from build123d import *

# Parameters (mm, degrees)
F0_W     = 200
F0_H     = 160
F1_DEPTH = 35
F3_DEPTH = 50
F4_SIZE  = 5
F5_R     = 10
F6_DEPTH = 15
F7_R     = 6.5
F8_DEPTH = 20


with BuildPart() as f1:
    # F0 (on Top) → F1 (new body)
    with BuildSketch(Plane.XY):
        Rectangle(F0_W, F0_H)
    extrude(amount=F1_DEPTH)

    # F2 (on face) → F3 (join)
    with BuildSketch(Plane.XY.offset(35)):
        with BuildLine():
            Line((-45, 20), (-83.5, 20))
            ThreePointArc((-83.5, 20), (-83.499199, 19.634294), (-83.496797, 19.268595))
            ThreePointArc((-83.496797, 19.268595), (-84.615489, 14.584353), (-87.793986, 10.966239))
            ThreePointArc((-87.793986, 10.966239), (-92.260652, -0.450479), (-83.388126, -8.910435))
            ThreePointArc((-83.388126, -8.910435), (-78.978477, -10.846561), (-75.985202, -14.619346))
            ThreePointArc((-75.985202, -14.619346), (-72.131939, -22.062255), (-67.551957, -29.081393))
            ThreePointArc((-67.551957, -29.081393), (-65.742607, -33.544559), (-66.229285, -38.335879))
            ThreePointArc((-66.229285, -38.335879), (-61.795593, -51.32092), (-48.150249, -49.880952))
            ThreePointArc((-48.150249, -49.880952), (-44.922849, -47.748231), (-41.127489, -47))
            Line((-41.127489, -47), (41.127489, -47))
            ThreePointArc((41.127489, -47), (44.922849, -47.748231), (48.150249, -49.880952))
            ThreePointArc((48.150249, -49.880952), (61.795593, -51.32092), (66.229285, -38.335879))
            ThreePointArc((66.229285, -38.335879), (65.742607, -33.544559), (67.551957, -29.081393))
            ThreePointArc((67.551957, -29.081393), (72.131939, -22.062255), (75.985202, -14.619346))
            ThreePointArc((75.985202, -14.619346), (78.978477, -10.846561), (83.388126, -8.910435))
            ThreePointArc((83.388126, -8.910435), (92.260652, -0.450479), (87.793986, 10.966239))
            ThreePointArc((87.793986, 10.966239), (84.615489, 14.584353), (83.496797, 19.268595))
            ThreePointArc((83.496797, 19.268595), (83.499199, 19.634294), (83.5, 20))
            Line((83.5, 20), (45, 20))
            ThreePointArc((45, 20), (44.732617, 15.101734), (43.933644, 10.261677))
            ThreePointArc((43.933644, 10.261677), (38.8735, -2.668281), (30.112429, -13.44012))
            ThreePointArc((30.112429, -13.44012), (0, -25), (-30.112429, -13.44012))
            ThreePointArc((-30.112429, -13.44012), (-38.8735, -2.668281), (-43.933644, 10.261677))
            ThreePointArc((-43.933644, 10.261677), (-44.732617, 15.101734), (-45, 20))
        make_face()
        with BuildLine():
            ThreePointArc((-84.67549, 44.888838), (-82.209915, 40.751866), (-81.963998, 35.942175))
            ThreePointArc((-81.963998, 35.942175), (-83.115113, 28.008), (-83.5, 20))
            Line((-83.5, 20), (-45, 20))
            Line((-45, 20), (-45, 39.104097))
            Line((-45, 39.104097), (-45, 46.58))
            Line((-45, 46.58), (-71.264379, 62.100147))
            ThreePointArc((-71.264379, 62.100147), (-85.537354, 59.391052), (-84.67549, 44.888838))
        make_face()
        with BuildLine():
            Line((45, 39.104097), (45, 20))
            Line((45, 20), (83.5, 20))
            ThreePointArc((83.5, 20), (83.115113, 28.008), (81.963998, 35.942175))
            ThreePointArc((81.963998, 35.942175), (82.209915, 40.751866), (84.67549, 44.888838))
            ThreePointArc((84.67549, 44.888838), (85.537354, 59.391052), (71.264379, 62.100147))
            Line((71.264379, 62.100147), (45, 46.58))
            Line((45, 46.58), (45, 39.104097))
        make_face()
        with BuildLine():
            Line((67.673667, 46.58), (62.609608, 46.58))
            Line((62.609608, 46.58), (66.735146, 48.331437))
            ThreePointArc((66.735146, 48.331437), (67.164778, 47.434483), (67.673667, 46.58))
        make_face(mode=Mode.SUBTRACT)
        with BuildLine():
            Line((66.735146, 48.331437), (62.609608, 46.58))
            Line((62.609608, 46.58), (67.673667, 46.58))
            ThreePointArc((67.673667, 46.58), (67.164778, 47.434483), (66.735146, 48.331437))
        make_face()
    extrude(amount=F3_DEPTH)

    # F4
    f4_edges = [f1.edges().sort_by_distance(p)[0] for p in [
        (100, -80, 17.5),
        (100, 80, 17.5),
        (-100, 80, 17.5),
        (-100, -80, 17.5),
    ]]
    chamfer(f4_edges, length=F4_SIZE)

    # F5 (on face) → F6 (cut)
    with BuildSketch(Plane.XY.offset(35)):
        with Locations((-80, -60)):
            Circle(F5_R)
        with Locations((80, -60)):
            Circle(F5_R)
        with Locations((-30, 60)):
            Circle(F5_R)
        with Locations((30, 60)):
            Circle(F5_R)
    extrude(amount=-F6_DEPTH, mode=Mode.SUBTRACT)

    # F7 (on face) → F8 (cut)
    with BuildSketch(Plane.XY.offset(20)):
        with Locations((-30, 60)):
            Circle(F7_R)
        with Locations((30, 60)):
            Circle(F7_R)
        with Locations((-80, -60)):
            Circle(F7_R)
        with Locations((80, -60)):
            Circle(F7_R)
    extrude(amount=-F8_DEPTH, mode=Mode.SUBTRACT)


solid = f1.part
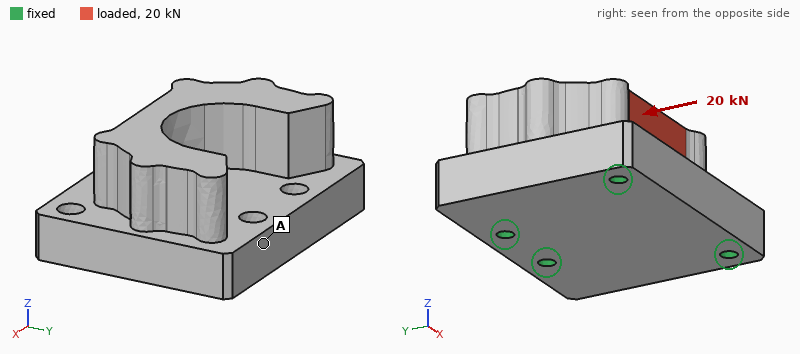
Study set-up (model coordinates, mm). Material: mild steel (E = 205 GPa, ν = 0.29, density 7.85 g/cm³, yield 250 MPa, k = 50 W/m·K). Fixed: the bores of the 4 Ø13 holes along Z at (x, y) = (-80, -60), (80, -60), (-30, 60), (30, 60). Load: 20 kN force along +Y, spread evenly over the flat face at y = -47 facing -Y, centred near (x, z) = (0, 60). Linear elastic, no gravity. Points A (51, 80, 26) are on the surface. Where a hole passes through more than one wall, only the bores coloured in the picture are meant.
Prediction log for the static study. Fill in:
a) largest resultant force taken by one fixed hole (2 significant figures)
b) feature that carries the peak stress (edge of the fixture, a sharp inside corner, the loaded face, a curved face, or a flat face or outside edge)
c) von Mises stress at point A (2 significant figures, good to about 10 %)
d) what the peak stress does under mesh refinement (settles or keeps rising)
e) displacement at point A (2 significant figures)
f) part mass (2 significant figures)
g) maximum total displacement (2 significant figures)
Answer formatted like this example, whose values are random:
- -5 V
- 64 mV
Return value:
- 7.1 kN
- edge of the fixture
- 3.7 MPa
- keeps rising
- 2.0 µm
- 13 kg
- 12 µm
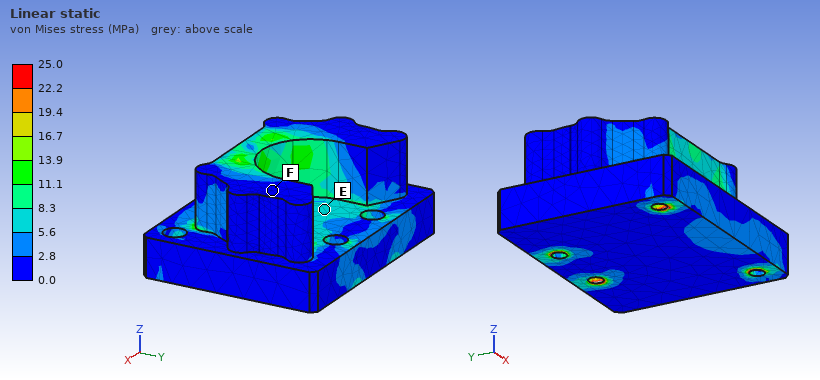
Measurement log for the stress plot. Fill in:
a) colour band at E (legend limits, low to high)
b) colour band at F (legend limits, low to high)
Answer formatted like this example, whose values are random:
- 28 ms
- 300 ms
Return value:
- 5.6 to 8.3 MPa
- 0.0 to 2.8 MPa
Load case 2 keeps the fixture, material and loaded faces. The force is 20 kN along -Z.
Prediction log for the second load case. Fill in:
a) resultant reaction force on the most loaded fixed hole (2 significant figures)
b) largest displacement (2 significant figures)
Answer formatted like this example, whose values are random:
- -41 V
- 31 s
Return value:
- 10 kN
- 12 µm
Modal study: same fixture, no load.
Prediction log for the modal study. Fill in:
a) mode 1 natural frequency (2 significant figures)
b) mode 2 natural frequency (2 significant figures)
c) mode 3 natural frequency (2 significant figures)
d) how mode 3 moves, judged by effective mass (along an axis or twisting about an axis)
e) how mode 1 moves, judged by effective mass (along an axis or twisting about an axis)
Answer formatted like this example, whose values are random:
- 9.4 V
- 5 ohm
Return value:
- 3500 Hz
- 3800 Hz
- 4300 Hz
- along Z
- along X
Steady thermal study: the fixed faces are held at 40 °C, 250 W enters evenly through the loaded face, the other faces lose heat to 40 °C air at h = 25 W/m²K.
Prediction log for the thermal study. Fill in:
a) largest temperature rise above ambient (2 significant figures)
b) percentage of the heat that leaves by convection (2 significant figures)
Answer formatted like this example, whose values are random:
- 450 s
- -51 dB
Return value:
- 78 K
- 23 %
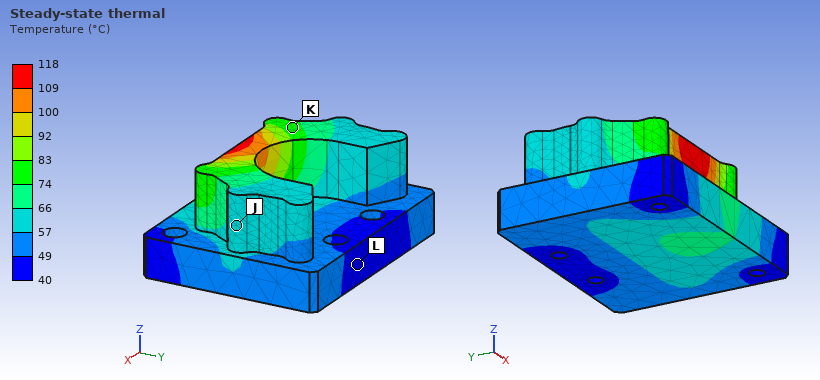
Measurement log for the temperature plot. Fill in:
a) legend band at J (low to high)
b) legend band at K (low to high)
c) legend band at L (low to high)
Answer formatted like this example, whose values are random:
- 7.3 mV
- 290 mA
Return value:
- 57 to 66 °C
- 74 to 83 °C
- 40 to 49 °C
